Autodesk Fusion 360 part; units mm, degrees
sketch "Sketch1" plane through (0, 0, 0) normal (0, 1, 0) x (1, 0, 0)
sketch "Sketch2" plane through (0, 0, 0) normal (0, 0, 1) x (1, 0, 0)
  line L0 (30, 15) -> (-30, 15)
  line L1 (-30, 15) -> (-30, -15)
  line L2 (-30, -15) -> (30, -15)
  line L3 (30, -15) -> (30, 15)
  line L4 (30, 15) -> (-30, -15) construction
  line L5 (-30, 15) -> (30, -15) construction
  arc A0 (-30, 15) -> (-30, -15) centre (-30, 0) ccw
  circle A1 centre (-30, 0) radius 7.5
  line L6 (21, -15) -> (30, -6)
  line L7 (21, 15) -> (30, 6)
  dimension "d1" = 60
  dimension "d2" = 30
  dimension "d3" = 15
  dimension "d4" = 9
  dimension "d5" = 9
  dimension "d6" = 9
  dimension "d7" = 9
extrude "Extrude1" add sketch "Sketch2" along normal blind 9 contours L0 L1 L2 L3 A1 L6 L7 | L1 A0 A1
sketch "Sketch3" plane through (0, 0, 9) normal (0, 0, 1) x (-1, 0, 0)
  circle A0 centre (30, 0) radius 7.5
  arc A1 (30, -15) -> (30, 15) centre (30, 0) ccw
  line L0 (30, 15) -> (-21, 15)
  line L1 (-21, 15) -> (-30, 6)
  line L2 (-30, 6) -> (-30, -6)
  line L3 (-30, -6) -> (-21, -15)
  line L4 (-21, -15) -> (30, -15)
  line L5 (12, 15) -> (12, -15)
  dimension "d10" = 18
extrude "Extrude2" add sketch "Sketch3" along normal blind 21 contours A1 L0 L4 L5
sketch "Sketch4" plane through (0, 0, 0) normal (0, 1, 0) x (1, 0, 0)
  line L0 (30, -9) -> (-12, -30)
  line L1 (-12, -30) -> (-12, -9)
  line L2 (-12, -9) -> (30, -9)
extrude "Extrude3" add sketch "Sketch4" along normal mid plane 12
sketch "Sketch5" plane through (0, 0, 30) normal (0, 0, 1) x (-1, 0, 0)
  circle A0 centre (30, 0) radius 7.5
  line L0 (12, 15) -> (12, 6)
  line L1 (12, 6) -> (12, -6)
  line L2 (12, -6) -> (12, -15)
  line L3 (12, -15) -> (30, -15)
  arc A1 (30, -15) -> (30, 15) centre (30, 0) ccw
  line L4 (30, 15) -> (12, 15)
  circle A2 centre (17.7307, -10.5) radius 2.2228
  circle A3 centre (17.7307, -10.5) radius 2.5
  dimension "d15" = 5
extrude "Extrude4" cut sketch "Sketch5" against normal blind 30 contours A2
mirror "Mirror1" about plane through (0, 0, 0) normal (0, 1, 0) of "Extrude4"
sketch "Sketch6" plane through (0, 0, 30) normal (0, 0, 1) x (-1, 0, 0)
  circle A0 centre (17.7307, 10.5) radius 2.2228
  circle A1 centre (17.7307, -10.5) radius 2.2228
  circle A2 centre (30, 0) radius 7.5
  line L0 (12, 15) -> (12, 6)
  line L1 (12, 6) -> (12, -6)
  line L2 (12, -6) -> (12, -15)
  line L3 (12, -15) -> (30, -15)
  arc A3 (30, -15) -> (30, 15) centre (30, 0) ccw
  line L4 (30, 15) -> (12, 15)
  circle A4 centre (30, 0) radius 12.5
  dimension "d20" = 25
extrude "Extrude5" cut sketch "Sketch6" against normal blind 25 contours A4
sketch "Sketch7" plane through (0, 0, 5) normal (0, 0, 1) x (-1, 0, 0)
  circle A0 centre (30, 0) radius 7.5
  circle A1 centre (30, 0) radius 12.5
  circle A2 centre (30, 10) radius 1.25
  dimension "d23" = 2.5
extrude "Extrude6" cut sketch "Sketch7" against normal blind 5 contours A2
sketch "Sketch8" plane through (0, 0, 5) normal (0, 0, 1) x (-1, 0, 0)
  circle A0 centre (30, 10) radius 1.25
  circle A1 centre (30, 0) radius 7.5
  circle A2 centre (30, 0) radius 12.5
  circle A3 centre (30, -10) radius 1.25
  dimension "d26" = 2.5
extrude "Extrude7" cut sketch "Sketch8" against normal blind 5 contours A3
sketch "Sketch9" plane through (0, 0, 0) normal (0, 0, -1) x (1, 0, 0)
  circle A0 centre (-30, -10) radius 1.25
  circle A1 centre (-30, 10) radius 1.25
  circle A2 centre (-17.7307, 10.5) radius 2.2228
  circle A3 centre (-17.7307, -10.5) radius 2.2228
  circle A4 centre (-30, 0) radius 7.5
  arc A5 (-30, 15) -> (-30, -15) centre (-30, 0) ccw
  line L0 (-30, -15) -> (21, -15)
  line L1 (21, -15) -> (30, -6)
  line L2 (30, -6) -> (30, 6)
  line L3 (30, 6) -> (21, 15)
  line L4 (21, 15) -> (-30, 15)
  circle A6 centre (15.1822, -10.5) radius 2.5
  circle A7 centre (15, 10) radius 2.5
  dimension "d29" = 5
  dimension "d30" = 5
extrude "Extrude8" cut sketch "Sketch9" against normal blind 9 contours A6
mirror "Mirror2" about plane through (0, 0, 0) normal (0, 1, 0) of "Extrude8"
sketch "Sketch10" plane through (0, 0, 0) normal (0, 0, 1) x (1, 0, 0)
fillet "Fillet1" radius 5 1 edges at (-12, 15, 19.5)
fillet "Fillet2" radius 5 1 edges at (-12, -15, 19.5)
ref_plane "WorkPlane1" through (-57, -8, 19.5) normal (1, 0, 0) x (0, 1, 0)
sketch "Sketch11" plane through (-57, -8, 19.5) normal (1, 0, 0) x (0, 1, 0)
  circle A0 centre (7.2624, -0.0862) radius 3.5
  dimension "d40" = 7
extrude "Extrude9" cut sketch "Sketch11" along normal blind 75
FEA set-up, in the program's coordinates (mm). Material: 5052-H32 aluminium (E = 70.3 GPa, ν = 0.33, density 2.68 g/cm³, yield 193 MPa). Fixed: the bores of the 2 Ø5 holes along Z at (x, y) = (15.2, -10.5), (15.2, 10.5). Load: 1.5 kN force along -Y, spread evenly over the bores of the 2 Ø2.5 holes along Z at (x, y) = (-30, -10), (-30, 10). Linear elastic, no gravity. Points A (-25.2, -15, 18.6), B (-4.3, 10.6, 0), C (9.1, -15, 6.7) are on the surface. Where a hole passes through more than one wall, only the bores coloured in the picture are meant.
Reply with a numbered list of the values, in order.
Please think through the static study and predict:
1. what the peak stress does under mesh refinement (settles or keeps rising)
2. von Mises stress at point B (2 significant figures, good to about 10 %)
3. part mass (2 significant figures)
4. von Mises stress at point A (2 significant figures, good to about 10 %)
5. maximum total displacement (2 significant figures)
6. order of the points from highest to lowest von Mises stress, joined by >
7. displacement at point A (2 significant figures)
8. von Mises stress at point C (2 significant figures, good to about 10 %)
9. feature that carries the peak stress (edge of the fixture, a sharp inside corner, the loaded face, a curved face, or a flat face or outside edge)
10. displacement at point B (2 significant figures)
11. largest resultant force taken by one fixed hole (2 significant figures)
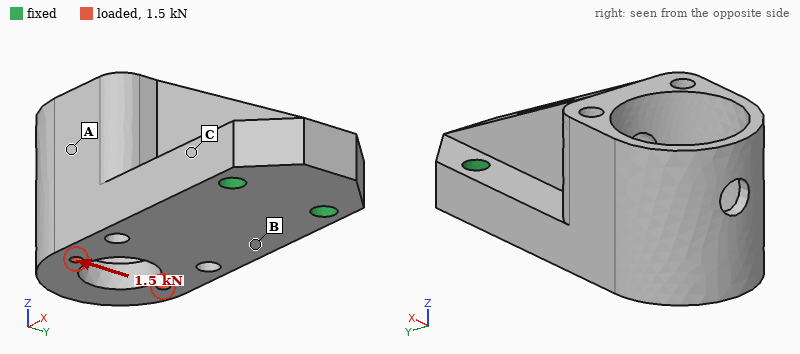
1. keeps rising
2. 22 MPa
3. 72 g
4. 9.5 MPa
5. 70 µm
6. C > B > A
7. 35 µm
8. 38 MPa
9. edge of the fixture
10. 14 µm
11. 3.0 kN
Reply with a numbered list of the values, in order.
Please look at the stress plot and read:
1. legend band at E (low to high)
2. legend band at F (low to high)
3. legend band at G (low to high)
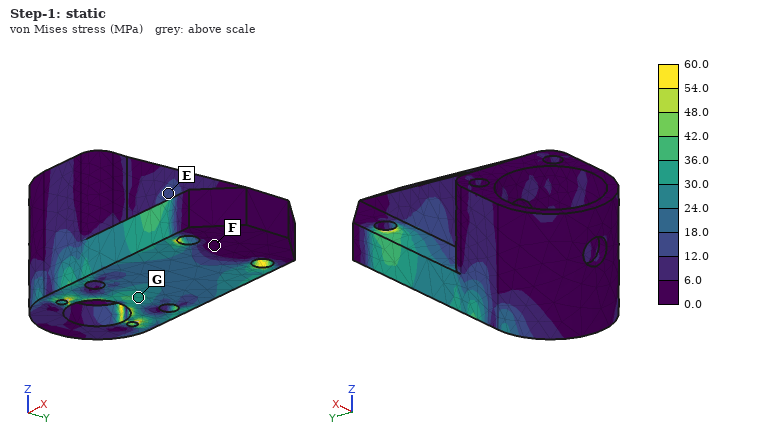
1. 12.0 to 18.0 MPa
2. 0.0 to 6.0 MPa
3. 30.0 to 36.0 MPa
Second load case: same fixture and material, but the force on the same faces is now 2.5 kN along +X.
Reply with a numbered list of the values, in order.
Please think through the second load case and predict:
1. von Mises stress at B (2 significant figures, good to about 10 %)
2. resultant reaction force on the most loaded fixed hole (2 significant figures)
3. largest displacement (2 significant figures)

1. 15 MPa
2. 1.3 kN
3. 36 µm
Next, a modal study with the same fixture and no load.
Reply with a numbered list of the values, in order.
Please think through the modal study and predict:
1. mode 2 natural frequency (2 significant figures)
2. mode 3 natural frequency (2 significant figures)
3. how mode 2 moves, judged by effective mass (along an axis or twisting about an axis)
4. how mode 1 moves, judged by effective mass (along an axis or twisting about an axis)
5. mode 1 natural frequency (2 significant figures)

1. 4900 Hz
2. 7300 Hz
3. along Y
4. along Z
5. 2700 Hz
